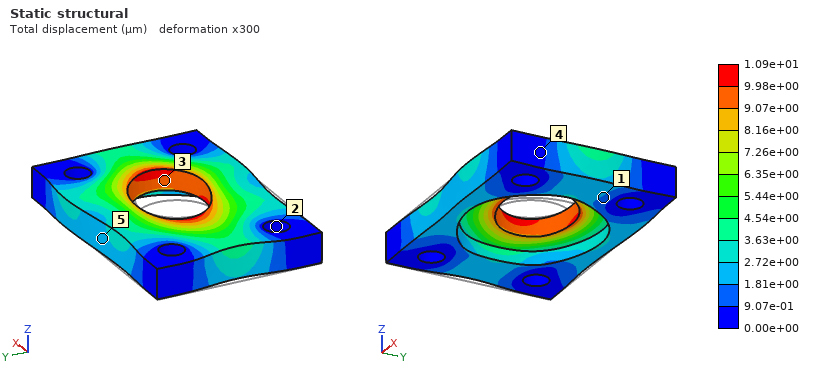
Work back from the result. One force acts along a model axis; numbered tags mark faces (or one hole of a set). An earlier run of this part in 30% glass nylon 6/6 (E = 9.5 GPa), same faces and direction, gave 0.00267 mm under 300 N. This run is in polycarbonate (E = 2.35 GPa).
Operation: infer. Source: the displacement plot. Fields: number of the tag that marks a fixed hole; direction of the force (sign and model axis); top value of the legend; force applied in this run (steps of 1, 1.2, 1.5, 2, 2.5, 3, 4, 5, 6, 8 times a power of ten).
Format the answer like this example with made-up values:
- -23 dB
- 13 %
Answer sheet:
- 2
- +X
- 1.09e+01 µm
- 300 N
